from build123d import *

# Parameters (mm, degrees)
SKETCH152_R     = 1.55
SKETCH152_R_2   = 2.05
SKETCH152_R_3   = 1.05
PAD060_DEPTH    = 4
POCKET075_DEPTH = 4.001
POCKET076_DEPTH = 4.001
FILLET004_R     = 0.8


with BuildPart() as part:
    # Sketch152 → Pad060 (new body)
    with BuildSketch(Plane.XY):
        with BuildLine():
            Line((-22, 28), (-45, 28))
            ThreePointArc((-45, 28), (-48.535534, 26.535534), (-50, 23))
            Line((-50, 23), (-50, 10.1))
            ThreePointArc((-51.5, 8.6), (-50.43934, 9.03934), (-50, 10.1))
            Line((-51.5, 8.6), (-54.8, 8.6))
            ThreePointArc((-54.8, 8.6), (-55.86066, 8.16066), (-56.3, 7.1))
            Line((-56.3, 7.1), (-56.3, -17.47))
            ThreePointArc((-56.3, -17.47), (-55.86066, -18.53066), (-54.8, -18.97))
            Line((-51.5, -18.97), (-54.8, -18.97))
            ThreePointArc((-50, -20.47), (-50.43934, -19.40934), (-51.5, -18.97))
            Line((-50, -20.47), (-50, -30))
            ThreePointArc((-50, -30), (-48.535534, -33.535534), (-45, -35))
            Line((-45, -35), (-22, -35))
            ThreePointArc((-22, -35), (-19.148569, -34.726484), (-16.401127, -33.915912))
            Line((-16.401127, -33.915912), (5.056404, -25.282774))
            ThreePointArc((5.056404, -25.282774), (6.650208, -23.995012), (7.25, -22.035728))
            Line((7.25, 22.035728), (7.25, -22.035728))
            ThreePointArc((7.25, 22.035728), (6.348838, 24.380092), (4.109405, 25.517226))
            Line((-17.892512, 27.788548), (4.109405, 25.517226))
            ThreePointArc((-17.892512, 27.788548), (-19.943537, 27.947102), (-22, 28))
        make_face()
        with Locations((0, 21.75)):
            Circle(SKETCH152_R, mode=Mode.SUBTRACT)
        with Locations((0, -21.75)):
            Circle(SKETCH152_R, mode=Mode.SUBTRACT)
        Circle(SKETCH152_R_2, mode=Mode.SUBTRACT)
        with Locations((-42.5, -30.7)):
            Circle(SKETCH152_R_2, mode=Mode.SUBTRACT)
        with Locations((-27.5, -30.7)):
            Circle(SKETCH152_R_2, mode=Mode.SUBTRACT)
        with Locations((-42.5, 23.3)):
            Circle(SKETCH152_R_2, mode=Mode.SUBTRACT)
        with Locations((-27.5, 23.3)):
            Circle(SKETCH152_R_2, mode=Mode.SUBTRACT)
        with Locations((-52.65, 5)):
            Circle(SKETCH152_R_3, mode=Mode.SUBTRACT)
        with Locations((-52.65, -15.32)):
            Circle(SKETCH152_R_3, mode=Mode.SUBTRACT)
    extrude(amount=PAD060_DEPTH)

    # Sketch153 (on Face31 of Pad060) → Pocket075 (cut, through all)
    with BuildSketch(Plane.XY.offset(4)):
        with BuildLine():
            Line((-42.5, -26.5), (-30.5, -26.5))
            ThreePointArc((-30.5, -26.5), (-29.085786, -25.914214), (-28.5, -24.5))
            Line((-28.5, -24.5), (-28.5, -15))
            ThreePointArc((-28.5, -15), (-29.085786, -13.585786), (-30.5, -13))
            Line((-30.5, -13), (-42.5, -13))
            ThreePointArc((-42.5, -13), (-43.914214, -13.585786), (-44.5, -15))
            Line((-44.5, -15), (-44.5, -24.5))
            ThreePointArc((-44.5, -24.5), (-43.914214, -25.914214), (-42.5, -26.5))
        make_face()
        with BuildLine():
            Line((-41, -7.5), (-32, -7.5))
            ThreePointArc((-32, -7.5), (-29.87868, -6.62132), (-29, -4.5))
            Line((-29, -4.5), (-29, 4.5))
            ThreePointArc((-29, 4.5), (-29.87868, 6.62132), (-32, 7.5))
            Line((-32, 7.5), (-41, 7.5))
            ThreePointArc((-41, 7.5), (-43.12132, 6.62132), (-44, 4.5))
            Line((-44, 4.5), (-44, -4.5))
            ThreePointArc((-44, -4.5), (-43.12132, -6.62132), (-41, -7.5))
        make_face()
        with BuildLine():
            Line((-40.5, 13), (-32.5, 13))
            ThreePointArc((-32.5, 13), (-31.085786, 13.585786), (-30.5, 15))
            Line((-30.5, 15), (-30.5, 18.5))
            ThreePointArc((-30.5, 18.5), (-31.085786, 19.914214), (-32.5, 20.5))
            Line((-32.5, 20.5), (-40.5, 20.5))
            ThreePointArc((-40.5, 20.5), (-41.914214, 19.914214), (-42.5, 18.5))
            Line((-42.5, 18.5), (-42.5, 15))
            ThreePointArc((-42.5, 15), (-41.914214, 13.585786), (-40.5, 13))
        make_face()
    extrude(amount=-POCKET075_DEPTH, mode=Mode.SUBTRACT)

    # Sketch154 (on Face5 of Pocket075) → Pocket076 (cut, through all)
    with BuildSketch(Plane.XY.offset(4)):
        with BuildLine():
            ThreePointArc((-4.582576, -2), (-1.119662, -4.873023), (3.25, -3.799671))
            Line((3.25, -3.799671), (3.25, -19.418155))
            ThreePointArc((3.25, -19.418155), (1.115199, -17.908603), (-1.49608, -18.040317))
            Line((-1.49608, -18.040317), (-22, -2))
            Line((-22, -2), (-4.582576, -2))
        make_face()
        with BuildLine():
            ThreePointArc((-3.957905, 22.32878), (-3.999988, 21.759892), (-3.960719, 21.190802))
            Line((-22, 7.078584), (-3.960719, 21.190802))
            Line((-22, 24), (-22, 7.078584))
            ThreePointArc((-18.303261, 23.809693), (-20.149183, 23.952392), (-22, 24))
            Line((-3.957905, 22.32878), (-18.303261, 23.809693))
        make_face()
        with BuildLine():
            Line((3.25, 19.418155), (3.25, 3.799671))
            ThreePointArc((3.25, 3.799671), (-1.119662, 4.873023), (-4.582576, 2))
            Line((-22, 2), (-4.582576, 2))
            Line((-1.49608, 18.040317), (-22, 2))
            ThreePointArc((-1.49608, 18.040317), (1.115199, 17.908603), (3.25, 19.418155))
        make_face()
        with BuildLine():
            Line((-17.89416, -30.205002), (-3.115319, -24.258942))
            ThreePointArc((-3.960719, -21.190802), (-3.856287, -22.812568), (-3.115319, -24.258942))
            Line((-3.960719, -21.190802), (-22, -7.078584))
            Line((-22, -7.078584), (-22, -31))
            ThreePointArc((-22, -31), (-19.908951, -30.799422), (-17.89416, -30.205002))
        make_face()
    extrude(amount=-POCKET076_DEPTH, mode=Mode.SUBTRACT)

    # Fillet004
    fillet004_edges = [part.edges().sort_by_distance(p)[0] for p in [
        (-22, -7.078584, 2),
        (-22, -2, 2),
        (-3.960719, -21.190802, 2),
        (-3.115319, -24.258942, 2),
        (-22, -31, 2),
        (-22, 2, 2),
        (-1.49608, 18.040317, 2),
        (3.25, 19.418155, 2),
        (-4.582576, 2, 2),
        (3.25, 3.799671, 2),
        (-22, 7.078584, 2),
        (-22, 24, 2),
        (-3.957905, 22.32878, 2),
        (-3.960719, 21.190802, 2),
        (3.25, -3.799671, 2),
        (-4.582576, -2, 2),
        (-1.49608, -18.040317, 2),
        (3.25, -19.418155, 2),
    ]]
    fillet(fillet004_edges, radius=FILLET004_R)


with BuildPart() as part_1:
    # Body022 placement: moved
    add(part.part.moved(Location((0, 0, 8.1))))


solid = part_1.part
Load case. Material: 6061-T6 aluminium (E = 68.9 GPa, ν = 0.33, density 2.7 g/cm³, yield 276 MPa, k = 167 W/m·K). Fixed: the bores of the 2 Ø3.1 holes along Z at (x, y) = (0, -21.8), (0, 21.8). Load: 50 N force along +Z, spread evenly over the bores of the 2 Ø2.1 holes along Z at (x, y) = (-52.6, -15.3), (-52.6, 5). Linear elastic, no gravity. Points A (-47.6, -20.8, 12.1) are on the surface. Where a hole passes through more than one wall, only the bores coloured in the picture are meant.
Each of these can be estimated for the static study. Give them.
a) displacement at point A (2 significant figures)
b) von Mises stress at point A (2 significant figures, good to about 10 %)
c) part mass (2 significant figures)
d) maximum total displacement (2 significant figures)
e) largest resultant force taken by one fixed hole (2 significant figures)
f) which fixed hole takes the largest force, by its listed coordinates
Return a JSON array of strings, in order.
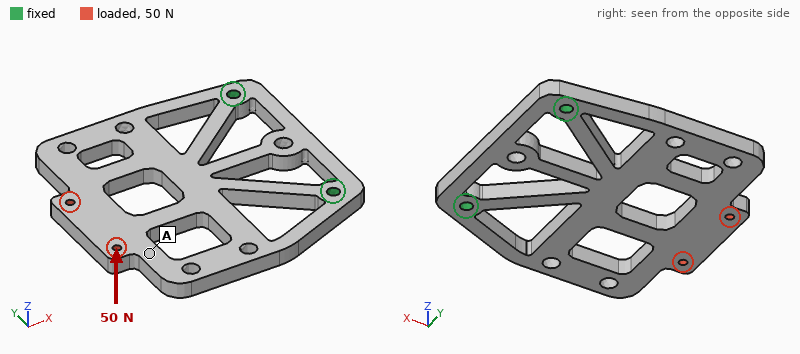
["0.35 mm", "9.1 MPa", "23 g", "0.44 mm", "29 N", "(0, -21.8)"]
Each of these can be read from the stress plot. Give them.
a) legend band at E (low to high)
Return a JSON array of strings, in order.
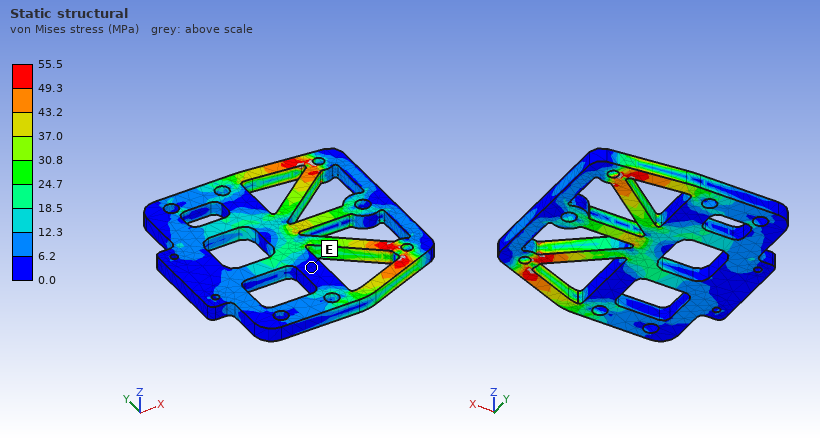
["0.0 to 6.2 MPa"]
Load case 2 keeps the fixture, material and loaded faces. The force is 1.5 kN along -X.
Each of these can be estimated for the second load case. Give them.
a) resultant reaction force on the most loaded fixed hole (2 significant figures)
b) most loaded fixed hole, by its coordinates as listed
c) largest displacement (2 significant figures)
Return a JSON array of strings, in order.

["940 N", "(0, -21.8)", "38 µm"]
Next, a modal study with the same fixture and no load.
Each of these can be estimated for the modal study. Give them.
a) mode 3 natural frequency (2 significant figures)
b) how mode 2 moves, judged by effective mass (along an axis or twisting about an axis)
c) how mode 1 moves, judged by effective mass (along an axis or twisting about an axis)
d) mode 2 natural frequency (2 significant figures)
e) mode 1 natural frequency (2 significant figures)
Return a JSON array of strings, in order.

["4300 Hz", "twisting about X", "along Z", "1900 Hz", "700 Hz"]
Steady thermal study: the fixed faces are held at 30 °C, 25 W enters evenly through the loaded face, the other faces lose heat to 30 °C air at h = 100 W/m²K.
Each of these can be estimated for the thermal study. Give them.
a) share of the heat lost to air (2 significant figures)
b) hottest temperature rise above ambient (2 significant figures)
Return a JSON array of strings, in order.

["64 %", "61 K"]
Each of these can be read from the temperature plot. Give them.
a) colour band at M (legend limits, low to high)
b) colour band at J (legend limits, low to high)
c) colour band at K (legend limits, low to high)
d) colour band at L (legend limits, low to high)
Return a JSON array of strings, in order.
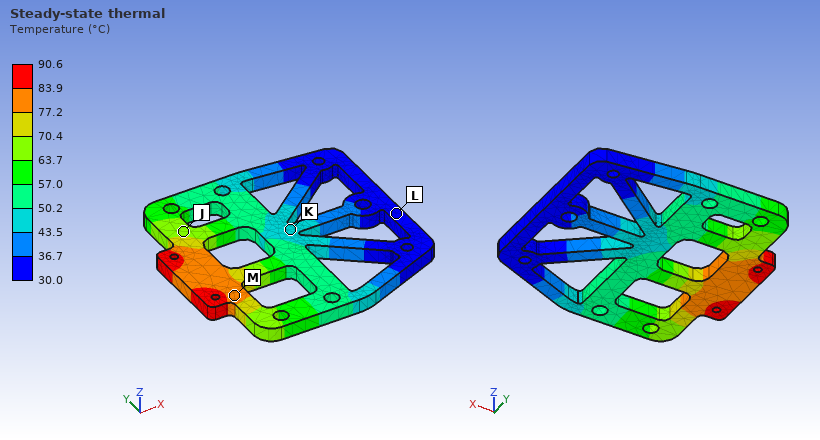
["77.2 to 83.9 °C", "63.7 to 70.4 °C", "43.5 to 50.2 °C", "30.0 to 36.7 °C"]
